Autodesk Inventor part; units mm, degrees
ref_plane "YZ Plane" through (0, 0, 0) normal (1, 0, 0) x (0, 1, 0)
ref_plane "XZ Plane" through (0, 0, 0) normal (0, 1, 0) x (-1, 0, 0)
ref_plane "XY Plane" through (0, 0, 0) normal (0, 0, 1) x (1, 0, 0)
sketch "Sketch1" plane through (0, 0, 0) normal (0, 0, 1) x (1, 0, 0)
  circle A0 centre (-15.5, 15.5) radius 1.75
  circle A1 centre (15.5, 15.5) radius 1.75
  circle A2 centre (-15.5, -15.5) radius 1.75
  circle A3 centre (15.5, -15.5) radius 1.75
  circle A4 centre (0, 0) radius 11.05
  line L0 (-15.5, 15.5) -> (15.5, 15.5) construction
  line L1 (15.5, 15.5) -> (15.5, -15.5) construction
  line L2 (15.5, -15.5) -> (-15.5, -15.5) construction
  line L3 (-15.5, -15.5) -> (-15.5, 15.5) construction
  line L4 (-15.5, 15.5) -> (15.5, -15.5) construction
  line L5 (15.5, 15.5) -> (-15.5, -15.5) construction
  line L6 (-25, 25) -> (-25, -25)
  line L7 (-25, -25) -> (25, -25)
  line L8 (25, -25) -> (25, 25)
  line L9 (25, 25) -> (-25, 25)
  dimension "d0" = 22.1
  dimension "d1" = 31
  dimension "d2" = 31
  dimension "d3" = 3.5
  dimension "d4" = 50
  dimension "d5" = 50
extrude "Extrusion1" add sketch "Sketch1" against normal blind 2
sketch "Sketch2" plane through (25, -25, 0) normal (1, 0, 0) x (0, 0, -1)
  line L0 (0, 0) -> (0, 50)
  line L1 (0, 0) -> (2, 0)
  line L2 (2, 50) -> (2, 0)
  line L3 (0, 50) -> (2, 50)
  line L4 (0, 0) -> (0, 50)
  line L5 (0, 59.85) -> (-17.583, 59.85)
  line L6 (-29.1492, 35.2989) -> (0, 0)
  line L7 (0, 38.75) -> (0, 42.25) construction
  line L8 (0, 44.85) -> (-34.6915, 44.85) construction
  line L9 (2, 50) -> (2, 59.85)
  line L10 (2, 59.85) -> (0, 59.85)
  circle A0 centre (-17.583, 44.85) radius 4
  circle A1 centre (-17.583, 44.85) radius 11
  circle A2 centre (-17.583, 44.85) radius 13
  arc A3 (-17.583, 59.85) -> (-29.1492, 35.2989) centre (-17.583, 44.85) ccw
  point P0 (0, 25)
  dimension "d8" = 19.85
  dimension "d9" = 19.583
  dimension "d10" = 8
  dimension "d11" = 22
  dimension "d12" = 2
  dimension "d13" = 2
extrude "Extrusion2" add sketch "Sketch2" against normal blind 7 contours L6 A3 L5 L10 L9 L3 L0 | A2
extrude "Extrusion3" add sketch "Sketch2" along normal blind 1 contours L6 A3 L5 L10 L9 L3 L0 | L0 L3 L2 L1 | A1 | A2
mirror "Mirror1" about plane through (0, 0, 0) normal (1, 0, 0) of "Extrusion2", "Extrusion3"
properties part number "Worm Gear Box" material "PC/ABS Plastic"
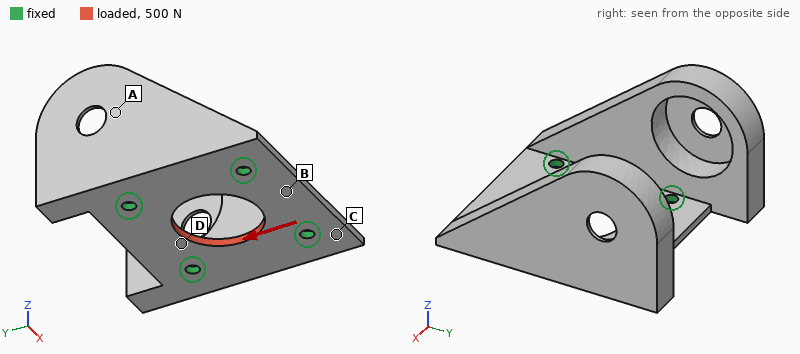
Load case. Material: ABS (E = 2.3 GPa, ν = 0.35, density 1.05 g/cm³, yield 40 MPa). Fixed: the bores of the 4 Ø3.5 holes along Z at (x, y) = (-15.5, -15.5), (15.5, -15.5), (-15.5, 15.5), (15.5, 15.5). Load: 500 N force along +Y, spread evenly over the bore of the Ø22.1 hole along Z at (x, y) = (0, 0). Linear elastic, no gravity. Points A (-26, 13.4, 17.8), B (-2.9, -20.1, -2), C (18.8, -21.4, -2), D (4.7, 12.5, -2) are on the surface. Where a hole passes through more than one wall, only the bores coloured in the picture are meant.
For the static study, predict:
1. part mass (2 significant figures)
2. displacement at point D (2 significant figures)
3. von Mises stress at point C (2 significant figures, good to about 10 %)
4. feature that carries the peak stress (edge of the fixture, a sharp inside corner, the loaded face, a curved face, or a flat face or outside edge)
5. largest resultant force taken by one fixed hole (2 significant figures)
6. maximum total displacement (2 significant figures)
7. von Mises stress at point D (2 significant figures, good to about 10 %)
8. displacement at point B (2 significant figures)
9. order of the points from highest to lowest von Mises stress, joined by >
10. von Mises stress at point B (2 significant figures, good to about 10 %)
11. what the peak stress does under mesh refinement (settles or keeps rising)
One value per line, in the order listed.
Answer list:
20 g
41 µm
1.5 MPa
edge of the fixture
130 N
50 µm
3.2 MPa
39 µm
D > B > C > A
2.5 MPa
keeps rising
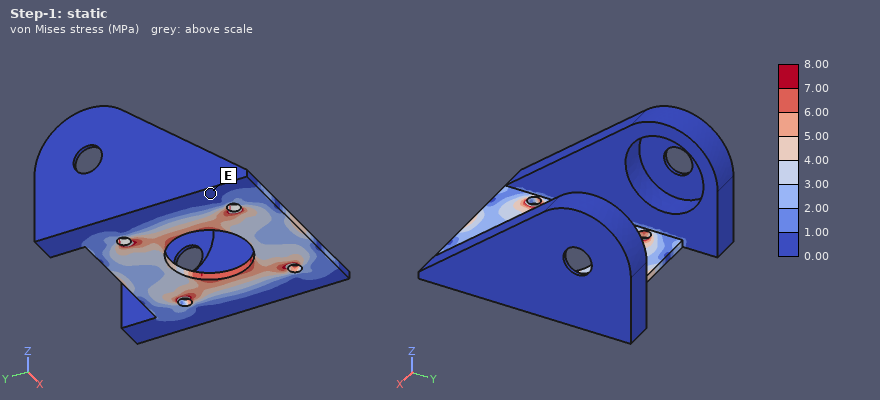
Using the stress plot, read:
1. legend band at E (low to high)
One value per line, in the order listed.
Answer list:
0.00 to 1.00 MPa
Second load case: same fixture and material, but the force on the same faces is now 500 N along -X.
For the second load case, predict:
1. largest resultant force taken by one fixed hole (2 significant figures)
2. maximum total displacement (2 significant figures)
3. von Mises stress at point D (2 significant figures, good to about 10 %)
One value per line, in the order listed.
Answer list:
130 N
44 µm
4.4 MPa
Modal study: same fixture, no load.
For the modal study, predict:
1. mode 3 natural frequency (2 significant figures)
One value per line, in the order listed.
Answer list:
1900 Hz
